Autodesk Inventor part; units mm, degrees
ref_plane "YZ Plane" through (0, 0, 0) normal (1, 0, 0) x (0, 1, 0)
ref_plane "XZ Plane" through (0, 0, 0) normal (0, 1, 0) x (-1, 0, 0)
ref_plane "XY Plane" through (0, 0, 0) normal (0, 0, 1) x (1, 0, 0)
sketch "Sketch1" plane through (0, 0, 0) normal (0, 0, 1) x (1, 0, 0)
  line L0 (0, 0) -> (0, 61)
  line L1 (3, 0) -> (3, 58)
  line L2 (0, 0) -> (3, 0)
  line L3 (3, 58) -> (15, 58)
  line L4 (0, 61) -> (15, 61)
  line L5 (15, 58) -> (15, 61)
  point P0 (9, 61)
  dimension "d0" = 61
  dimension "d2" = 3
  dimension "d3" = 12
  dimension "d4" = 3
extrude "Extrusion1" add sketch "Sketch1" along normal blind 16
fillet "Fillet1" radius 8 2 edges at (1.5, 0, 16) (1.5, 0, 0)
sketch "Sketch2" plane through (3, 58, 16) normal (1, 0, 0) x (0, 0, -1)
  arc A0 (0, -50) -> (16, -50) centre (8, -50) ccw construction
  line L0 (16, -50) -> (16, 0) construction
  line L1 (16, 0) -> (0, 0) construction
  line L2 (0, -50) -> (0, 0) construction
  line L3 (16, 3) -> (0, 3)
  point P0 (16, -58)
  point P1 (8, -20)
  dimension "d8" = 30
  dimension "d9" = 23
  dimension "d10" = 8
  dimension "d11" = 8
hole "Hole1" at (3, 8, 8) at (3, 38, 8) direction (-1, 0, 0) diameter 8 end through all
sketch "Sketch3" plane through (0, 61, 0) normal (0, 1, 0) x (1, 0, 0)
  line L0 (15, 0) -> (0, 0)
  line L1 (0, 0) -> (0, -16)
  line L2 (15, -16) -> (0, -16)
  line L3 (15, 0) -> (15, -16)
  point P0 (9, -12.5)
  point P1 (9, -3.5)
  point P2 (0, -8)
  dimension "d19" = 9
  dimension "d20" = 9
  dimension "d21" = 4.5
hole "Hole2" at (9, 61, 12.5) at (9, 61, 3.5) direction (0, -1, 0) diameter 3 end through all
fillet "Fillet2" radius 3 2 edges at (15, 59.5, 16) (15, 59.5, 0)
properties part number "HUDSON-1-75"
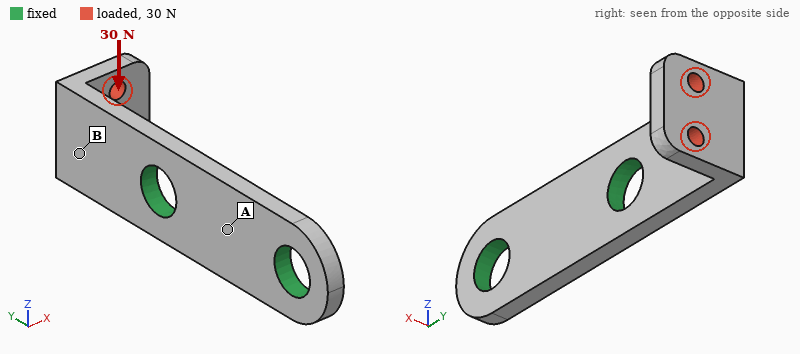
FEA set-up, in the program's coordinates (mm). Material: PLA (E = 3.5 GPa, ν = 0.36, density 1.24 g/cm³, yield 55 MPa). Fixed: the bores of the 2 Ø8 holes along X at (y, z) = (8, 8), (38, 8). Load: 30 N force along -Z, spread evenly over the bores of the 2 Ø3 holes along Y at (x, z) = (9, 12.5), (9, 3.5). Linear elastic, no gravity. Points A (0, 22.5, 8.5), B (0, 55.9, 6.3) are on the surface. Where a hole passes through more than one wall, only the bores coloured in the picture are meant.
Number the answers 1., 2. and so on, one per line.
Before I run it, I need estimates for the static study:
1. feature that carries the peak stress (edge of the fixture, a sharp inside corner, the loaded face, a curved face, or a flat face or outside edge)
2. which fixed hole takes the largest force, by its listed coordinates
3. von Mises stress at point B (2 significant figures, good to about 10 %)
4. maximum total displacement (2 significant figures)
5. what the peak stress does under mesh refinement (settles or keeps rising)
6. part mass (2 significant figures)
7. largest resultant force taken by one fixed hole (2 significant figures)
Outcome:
1. edge of the fixture
2. (38, 8)
3. 5.2 MPa
4. 0.33 mm
5. keeps rising
6. 3.8 g
7. 34 N
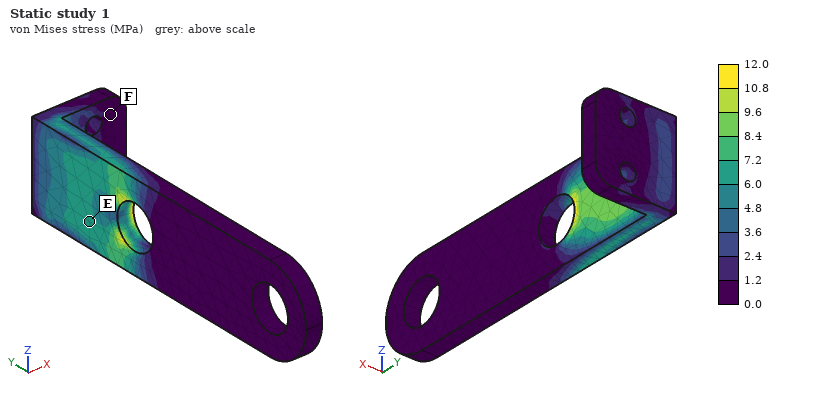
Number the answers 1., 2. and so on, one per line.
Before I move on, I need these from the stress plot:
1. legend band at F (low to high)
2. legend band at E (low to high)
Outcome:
1. 0.0 to 1.2 MPa
2. 6.0 to 7.2 MPa
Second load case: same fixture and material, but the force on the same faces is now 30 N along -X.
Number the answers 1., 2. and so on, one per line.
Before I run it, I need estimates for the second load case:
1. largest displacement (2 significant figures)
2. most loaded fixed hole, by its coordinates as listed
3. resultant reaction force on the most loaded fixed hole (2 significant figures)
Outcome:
1. 0.75 mm
2. (38, 8)
3. 30 N
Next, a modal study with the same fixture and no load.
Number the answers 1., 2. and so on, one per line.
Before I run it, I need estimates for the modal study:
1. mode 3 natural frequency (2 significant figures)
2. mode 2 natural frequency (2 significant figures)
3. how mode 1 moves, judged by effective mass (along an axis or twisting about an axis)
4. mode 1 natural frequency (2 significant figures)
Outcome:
1. 3500 Hz
2. 2000 Hz
3. along X
4. 1100 Hz
